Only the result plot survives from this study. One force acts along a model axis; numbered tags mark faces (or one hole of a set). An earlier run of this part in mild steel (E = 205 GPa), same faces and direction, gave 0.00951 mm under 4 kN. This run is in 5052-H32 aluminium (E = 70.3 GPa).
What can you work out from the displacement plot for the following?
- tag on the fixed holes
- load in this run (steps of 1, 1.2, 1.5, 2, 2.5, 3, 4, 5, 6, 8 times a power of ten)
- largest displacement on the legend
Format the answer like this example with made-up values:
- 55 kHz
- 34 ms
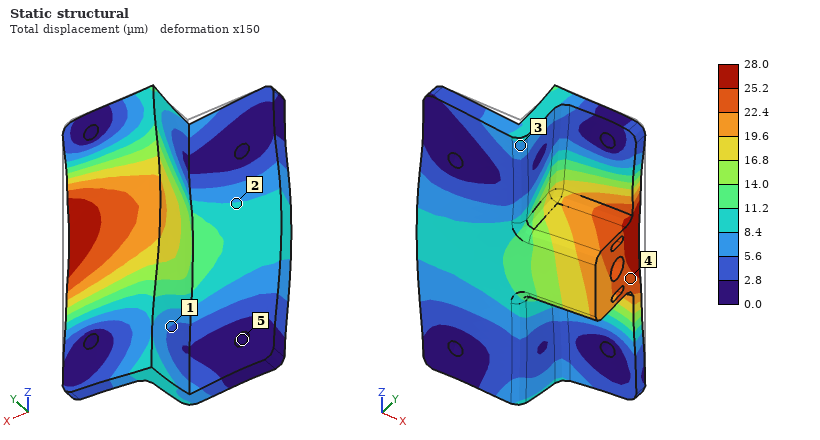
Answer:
- 5
- 4 kN
- 28.0 µm
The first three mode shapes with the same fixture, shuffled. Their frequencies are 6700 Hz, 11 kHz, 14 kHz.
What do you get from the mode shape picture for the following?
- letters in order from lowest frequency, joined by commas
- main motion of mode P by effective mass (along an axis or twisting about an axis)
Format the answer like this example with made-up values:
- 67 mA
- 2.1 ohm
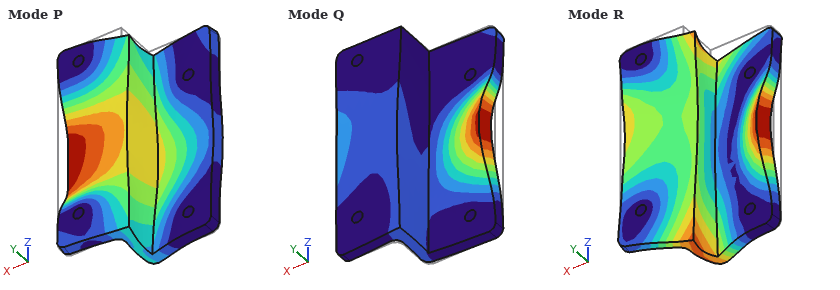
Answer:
- P, Q, R
- along Y
